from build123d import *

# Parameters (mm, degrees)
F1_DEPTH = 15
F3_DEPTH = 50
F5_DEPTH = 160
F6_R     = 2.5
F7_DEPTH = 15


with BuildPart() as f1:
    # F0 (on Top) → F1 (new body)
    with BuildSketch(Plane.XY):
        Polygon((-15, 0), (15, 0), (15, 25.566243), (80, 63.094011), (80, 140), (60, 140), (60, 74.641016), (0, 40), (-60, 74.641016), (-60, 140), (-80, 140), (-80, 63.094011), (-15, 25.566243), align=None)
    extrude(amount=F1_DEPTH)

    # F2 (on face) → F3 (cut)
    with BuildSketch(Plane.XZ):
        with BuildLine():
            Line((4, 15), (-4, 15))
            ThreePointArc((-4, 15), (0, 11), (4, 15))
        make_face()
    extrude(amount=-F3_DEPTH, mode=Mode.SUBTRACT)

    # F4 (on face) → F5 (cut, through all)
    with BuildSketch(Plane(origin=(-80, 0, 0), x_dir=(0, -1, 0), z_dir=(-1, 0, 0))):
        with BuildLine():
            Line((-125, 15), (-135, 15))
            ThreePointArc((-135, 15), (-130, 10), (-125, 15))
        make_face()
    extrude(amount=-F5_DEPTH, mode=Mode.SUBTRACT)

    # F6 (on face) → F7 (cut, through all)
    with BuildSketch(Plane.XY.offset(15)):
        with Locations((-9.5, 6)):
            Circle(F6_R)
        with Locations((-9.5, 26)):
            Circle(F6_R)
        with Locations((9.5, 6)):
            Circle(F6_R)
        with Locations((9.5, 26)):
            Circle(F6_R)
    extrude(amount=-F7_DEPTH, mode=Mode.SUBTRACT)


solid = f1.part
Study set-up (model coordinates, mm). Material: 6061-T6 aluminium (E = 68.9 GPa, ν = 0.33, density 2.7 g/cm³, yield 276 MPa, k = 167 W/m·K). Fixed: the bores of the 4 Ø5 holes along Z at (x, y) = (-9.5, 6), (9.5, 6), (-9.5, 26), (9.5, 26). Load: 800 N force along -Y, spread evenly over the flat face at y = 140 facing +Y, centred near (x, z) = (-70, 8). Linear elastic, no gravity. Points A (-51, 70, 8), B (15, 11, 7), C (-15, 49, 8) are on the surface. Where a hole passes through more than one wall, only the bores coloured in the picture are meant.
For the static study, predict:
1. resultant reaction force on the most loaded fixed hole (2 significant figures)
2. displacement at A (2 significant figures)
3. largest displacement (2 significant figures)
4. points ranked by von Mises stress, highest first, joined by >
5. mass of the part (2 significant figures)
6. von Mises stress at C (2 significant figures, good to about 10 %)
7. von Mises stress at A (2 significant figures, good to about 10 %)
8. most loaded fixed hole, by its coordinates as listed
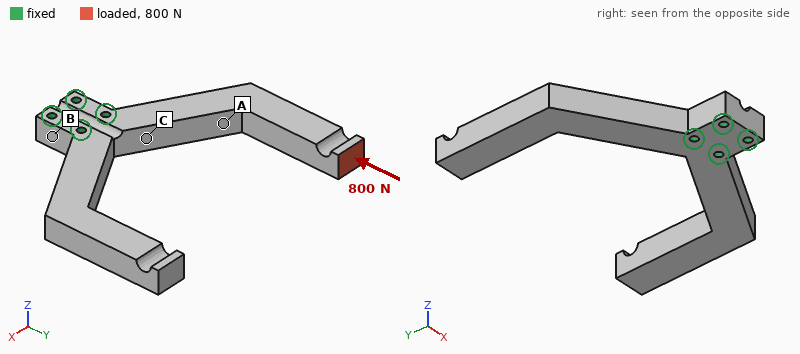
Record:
2.8 kN
0.12 mm
0.35 mm
C > A > B
260 g
39 MPa
9.7 MPa
(-9.5, 26)
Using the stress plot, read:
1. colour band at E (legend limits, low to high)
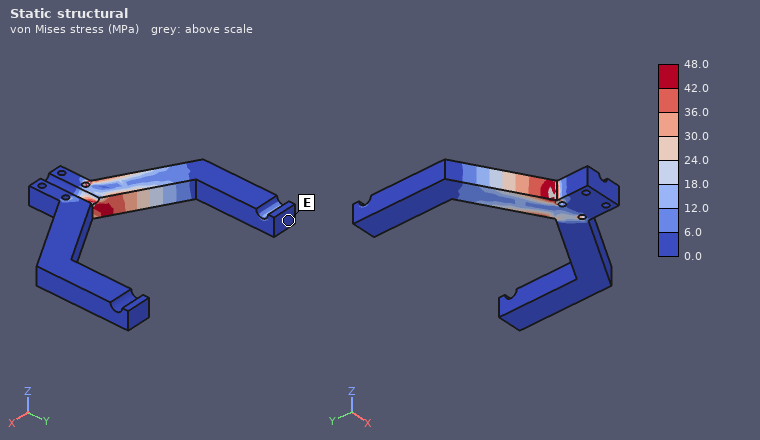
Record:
0.0 to 6.0 MPa
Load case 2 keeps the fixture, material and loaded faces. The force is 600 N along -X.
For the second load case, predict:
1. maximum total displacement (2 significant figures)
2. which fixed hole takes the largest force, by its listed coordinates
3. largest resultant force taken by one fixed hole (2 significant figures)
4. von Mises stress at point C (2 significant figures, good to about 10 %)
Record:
0.74 mm
(9.5, 26)
3.4 kN
62 MPa
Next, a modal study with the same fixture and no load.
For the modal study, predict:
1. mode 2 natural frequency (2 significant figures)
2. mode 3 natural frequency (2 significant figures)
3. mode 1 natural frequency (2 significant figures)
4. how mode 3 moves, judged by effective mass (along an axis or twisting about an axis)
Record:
640 Hz
820 Hz
640 Hz
along X
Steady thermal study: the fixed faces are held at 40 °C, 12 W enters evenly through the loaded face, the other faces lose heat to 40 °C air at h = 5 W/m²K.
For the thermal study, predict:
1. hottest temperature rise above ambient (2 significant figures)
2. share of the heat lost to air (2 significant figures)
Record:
34 K
7.1 %
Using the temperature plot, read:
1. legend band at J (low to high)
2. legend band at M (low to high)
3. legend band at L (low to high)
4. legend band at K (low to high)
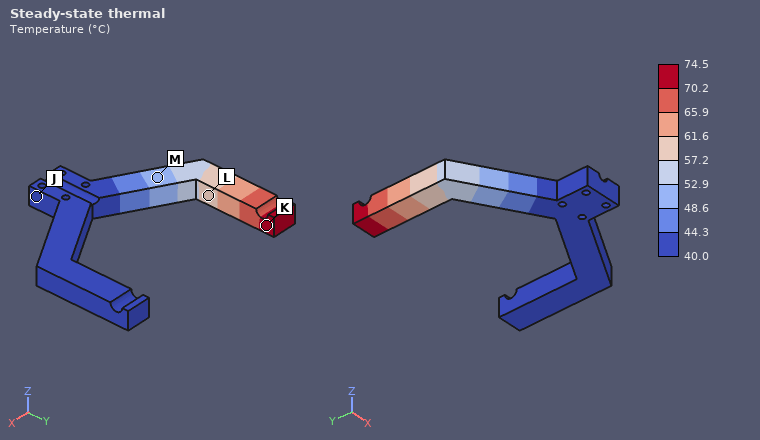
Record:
40.0 to 44.3 °C
48.6 to 52.9 °C
57.2 to 61.6 °C
70.2 to 74.5 °C
